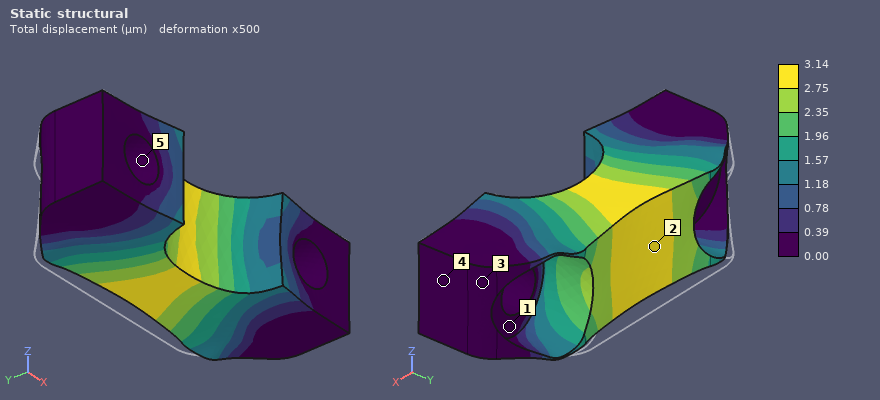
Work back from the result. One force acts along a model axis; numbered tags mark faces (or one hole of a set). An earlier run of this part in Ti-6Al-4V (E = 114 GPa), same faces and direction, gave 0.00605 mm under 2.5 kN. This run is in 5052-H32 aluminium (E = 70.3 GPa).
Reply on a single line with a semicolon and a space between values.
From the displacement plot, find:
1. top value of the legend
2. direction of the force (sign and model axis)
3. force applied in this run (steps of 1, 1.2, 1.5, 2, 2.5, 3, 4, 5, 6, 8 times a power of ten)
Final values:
3.14 µm; -Y; 800 N
